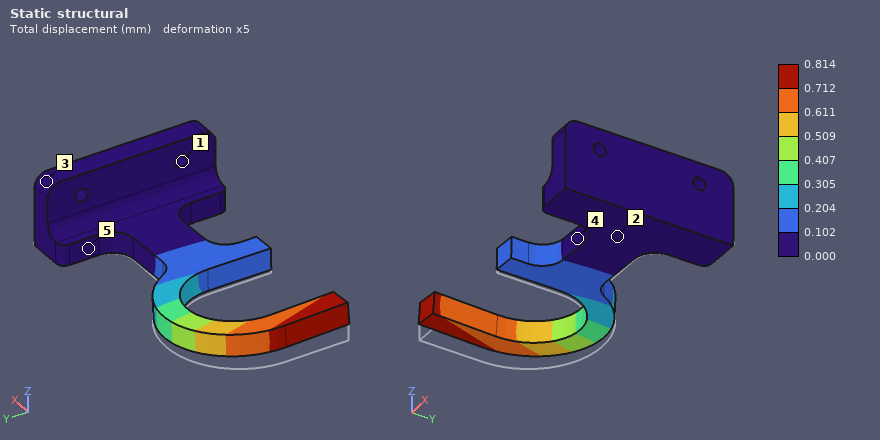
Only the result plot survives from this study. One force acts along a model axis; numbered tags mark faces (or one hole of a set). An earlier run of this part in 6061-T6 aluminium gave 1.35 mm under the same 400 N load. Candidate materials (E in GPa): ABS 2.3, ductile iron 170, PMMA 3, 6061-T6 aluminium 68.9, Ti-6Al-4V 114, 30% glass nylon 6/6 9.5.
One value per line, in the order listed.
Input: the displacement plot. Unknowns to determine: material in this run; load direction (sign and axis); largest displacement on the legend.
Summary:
Ti-6Al-4V
+Z
0.814 mm
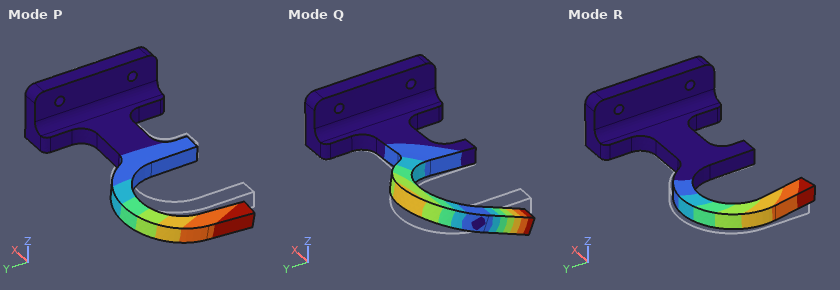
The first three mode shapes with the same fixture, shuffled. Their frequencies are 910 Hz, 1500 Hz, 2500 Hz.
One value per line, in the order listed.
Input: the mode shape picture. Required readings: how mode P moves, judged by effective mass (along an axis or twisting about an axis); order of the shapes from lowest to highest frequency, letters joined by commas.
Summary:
along Z
P, R, Q
